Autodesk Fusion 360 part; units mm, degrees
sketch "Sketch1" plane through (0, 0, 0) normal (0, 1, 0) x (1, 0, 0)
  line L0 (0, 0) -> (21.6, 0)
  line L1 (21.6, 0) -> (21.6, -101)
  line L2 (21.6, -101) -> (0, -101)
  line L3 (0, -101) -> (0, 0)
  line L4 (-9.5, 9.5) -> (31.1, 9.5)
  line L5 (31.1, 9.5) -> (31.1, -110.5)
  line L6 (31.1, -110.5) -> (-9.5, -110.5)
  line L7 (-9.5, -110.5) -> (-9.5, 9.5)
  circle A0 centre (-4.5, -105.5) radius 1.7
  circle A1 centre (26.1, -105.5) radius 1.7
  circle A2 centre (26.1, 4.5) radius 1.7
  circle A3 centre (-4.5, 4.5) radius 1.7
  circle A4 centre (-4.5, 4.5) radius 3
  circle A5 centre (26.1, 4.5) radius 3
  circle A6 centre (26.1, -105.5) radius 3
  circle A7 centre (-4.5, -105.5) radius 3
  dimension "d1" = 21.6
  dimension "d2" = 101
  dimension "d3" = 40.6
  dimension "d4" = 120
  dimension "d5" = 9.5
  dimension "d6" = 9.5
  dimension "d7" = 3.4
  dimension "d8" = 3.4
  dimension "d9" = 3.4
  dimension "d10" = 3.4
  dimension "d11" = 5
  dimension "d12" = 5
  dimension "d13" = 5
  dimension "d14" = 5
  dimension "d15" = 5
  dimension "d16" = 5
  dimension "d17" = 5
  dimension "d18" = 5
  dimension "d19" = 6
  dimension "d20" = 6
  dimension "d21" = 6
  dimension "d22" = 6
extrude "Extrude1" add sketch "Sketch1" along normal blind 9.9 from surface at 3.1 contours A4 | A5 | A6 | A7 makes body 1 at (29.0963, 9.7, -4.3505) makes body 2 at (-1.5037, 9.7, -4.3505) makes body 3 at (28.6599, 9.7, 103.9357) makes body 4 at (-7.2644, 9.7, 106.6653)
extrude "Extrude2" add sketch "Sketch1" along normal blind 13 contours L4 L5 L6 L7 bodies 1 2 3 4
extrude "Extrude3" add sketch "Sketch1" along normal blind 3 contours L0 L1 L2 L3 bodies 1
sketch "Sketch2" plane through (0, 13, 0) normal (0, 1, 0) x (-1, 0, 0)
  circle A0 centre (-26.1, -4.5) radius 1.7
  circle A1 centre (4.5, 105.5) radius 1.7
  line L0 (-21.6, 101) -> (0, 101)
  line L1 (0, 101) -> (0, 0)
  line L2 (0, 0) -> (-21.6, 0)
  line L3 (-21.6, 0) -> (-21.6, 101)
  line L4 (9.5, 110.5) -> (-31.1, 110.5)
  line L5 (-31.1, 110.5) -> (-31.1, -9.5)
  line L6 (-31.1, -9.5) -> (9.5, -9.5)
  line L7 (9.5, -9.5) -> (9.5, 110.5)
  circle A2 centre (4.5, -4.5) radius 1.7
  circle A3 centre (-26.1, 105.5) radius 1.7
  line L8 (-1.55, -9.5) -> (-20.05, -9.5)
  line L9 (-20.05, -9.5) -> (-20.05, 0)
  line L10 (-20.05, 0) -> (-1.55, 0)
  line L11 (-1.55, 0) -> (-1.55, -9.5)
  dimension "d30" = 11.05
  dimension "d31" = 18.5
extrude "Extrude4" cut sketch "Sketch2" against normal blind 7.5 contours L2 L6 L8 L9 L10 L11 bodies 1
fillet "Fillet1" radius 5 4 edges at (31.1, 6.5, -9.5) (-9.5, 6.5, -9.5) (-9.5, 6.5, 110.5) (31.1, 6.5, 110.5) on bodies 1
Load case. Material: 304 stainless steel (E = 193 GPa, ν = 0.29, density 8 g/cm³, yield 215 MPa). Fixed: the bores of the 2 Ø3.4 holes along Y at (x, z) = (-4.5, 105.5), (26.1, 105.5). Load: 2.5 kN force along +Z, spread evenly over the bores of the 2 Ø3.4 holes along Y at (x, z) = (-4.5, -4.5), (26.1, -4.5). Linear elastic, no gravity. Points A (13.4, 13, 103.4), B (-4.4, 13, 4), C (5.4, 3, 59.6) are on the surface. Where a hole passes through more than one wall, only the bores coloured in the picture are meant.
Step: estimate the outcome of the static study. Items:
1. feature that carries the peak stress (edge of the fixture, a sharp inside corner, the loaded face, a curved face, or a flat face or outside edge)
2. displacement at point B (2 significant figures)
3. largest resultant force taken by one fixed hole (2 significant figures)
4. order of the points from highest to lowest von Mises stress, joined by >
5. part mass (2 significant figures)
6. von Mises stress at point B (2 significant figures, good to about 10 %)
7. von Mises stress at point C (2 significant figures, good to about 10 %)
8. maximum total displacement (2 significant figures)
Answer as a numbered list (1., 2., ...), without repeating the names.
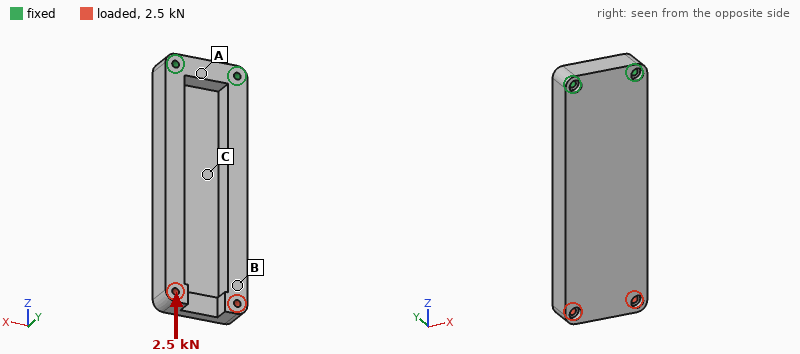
1. the loaded face
2. 34 µm
3. 1.3 kN
4. B > C > A
5. 310 g
6. 17 MPa
7. 4.6 MPa
8. 44 µm
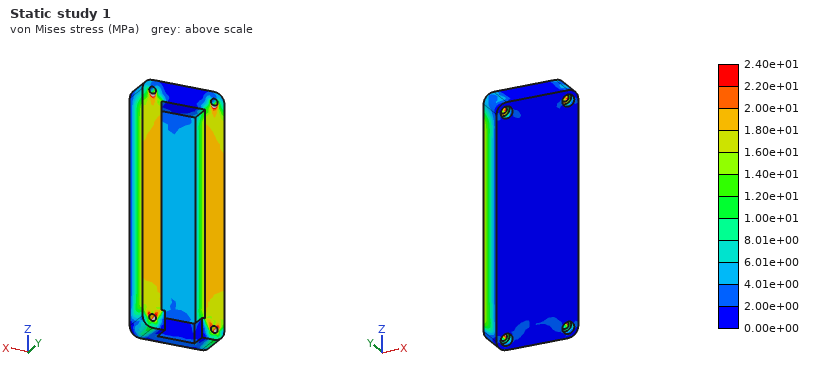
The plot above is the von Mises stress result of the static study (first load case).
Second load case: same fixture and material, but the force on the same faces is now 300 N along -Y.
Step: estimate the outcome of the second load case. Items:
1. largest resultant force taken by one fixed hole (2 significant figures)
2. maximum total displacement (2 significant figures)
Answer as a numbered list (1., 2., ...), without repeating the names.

1. 190 N
2. 0.18 mm
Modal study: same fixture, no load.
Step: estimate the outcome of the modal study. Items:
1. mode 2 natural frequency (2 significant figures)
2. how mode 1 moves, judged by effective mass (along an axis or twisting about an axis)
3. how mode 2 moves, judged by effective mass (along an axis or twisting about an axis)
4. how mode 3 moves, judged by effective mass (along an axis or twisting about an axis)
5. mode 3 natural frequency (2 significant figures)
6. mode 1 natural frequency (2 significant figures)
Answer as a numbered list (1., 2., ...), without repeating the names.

1. 1700 Hz
2. along Y
3. along X
4. along X
5. 2800 Hz
6. 720 Hz
